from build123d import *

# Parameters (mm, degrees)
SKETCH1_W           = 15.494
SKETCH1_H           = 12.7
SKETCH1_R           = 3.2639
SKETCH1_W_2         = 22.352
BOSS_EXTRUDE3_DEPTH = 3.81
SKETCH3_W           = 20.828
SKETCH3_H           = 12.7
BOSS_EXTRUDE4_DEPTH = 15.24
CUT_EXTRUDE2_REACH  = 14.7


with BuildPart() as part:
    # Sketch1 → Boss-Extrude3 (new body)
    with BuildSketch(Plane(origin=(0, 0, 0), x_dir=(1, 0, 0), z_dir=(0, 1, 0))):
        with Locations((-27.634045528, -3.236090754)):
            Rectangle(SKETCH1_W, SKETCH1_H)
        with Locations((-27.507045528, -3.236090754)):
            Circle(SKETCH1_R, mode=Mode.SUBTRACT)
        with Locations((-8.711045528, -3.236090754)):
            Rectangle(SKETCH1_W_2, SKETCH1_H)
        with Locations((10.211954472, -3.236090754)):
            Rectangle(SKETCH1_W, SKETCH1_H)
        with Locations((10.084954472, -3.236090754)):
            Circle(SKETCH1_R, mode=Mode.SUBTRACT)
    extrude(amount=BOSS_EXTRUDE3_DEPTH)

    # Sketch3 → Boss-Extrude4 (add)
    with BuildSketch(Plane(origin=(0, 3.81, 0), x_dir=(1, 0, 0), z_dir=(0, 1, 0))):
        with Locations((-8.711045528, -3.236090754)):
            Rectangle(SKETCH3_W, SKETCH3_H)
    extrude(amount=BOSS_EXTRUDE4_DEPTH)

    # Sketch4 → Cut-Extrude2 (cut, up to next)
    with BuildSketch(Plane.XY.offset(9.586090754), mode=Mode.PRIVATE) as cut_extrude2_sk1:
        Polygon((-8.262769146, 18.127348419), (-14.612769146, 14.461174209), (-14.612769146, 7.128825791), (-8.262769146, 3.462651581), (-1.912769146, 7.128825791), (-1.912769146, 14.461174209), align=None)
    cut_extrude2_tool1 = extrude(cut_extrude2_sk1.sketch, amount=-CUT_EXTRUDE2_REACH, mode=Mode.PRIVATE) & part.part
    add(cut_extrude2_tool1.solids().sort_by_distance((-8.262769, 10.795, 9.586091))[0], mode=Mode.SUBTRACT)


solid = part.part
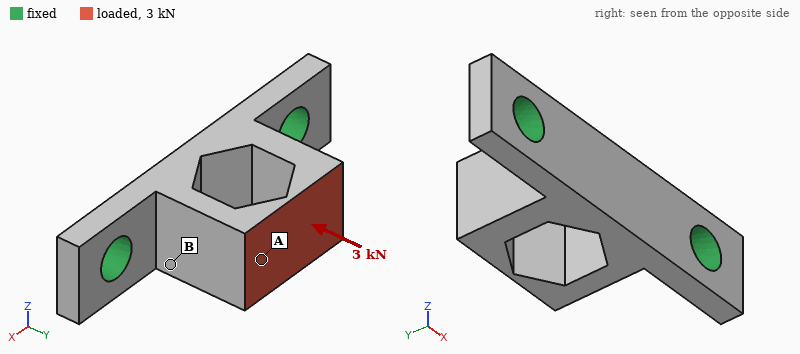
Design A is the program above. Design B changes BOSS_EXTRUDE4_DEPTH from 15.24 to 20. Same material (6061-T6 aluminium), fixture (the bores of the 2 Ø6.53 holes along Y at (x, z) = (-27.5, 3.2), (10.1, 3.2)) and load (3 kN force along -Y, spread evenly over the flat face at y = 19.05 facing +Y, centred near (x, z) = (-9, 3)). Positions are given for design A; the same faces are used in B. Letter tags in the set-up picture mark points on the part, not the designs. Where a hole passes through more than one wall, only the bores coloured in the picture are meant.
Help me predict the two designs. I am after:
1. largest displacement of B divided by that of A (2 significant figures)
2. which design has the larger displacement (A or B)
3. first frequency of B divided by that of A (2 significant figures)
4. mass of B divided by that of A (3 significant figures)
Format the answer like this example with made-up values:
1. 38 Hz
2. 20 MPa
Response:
1. 0.81
2. A
3. 0.63
4. 1.27
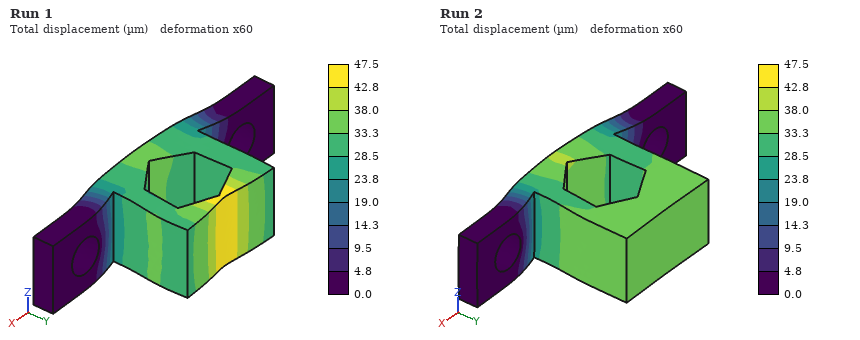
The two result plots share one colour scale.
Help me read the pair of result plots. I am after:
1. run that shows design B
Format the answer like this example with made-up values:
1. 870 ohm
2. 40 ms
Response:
1. Run 2
